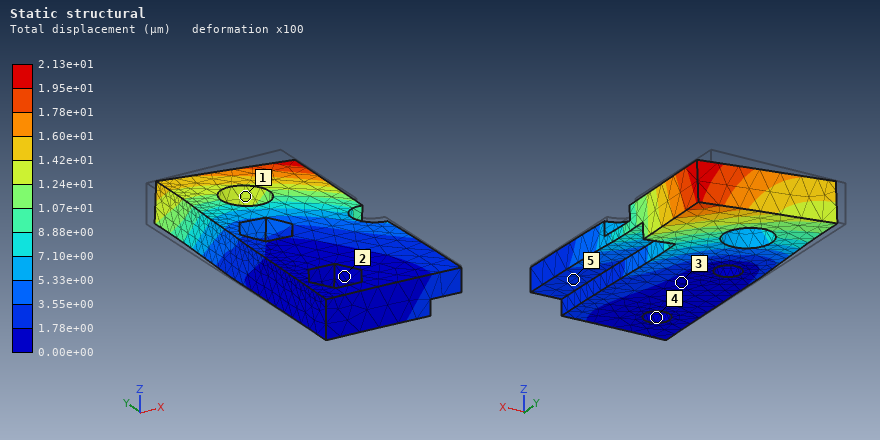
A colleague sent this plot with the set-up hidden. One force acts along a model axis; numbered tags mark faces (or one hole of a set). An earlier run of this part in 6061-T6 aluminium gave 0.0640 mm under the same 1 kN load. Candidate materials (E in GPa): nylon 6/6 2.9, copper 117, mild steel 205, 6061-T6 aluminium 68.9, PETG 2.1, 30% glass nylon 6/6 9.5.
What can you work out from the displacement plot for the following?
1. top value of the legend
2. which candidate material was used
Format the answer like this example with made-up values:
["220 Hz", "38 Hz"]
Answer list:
["2.13e+01 µm", "mild steel"]
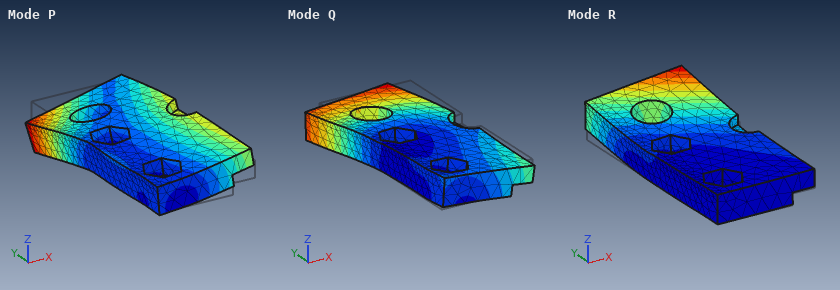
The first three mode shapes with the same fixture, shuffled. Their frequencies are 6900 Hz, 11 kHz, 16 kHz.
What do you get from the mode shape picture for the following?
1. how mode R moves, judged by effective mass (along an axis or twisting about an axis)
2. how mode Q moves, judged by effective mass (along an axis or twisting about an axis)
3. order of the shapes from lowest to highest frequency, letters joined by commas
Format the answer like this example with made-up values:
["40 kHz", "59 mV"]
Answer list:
["along Z", "along X", "R, P, Q"]
